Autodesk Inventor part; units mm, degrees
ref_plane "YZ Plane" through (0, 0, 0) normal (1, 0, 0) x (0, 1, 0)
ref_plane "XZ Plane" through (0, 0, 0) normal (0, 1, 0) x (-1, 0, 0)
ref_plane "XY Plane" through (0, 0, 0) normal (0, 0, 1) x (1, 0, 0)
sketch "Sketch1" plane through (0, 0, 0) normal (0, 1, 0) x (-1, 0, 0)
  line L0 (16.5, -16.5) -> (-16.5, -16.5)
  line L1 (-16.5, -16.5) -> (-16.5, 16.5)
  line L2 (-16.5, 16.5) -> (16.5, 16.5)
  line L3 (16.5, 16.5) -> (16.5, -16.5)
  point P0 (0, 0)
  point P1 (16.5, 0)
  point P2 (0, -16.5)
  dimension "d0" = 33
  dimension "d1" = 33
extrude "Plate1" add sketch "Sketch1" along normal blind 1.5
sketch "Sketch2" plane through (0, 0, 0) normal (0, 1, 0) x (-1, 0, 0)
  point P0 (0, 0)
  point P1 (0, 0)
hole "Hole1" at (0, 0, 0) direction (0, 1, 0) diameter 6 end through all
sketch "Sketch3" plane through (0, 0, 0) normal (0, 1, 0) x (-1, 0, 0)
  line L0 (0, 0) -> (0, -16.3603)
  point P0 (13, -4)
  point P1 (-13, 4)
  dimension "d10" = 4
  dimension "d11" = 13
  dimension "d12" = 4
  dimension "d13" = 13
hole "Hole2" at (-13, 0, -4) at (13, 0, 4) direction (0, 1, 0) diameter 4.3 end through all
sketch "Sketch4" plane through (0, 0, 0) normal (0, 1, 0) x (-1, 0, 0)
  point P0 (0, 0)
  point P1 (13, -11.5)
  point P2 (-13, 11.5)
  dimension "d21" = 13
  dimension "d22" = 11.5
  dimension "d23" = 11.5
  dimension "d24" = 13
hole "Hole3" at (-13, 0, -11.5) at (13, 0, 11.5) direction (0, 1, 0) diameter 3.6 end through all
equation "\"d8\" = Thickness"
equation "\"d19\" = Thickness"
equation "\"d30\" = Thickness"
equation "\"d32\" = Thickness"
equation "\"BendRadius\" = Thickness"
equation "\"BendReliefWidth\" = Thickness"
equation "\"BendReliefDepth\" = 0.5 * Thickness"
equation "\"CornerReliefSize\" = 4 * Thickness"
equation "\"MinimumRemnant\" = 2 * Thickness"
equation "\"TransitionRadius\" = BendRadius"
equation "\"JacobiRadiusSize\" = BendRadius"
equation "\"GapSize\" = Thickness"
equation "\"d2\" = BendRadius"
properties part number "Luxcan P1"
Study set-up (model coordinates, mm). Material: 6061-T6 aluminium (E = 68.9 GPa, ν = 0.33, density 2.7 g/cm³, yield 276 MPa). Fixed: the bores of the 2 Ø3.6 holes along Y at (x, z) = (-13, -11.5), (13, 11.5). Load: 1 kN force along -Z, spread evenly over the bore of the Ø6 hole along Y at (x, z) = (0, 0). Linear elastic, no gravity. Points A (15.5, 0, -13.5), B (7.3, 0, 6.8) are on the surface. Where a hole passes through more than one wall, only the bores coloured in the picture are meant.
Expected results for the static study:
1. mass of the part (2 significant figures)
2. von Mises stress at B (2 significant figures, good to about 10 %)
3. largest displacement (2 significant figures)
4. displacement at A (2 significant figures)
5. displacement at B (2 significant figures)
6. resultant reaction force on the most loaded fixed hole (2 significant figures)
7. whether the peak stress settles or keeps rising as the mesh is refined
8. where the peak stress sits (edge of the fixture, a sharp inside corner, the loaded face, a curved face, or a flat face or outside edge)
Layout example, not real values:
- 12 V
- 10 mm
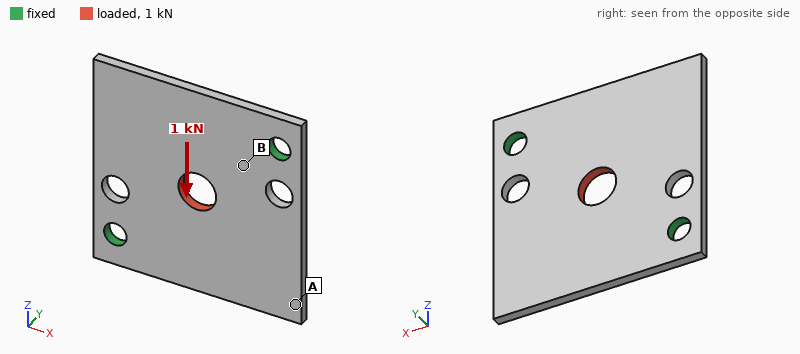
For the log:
- 4.1 g
- 28 MPa
- 13 µm
- 8.4 µm
- 7.0 µm
- 500 N
- keeps rising
- edge of the fixture
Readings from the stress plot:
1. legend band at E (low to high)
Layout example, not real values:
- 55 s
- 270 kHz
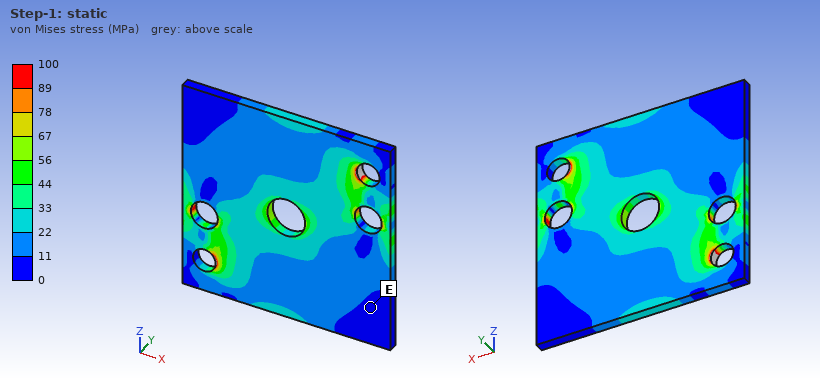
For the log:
- 0 to 11 MPa
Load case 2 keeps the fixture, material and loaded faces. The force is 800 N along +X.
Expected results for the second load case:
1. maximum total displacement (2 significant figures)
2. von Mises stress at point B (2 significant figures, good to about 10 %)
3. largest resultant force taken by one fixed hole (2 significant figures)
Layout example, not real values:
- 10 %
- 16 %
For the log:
- 9.0 µm
- 29 MPa
- 400 N
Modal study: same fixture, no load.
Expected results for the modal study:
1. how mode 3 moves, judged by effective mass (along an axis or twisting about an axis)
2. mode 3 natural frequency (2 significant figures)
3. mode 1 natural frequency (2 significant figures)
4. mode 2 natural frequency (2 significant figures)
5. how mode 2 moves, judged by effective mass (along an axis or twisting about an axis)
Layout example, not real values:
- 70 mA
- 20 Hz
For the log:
- along Y
- 8800 Hz
- 2600 Hz
- 3300 Hz
- along Y
